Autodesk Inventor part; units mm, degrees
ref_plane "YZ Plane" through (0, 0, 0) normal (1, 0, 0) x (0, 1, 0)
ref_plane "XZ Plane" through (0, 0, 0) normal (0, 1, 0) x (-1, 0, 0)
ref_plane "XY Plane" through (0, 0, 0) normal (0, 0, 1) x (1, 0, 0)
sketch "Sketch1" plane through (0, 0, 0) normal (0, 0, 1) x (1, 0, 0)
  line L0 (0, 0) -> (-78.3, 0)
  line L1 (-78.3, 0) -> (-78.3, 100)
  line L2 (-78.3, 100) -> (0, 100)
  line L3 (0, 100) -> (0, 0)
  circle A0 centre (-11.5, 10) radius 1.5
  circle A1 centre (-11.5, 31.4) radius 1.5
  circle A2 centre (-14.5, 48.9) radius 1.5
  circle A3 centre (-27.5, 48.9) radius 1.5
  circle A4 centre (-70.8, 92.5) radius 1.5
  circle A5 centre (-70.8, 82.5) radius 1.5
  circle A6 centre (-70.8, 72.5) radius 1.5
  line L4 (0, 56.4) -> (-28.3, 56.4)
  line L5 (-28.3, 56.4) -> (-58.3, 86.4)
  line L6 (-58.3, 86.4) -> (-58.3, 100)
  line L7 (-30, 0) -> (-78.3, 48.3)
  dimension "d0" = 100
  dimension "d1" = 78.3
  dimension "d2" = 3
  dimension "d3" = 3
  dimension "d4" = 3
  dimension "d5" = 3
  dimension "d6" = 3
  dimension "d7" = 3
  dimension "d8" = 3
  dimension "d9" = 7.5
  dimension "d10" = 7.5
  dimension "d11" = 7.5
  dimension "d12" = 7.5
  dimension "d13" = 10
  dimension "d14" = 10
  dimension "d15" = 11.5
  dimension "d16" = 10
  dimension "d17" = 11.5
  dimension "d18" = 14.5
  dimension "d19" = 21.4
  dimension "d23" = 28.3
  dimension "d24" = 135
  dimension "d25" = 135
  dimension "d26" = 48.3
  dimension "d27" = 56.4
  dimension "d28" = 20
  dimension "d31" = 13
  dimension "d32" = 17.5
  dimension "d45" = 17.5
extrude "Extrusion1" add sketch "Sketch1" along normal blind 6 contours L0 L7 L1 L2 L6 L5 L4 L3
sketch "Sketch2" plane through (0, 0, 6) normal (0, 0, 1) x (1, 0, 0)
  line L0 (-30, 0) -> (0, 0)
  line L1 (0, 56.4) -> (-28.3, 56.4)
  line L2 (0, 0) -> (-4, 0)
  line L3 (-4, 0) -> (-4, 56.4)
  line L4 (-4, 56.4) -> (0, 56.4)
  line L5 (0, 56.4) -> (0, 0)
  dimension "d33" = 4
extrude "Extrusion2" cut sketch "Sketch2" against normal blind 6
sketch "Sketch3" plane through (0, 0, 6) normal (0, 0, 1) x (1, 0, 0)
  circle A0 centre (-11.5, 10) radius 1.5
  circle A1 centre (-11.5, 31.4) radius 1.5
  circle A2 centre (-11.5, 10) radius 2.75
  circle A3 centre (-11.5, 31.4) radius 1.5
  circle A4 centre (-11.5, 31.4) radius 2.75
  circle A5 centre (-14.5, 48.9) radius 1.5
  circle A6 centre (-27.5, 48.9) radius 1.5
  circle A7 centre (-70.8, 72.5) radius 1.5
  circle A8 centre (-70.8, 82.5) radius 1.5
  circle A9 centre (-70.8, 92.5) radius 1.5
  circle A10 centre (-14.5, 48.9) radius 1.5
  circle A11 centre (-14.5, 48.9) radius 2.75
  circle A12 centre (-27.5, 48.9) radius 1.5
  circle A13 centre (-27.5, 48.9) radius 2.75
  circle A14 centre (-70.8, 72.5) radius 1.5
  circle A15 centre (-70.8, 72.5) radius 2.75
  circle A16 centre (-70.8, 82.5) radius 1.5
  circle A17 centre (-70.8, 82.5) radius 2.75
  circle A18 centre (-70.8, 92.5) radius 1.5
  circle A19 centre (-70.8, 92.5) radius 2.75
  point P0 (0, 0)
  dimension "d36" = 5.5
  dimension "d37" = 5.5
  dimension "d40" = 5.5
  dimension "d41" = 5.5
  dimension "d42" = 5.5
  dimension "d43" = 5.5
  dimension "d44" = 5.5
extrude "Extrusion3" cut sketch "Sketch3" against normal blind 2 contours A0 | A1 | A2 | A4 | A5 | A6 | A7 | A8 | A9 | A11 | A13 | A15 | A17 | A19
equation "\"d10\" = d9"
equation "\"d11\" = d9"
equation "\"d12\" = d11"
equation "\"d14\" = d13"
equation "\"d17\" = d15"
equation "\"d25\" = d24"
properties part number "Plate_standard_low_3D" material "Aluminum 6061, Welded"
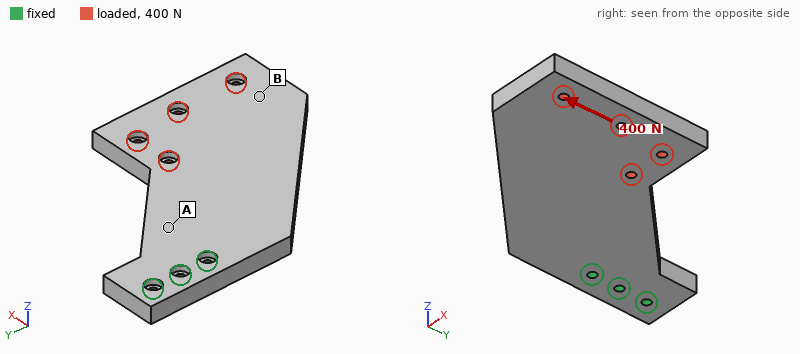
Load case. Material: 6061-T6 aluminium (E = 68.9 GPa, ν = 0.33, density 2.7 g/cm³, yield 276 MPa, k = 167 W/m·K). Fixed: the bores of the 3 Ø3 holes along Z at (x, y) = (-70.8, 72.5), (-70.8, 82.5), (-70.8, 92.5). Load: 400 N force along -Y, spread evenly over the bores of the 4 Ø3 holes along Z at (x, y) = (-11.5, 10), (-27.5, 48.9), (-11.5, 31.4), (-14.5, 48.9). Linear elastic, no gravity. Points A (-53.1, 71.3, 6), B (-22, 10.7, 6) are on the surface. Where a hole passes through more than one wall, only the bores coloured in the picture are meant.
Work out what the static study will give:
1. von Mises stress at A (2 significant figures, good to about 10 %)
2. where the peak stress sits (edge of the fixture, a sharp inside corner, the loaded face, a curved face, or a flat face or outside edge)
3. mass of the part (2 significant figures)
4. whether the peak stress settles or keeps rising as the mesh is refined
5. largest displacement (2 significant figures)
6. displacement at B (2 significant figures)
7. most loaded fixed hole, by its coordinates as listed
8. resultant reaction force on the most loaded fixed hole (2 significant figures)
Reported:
10 MPa
edge of the fixture
69 g
keeps rising
0.10 mm
0.079 mm
(-70.8, 72.5)
1.2 kN
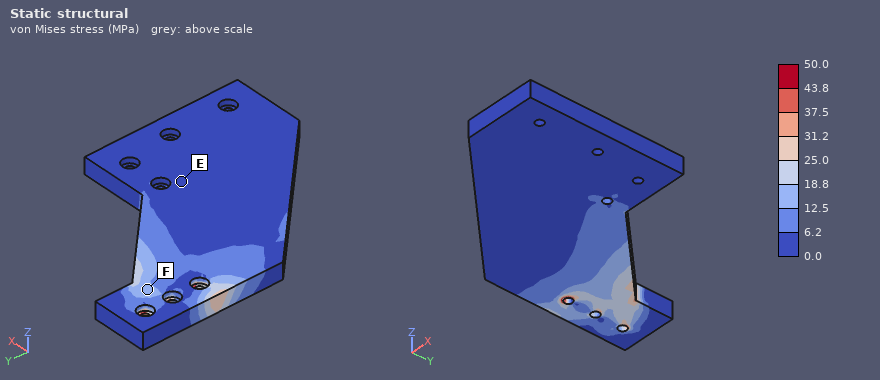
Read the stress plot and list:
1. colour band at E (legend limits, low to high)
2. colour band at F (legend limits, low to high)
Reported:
0.0 to 6.2 MPa
12.5 to 18.8 MPa
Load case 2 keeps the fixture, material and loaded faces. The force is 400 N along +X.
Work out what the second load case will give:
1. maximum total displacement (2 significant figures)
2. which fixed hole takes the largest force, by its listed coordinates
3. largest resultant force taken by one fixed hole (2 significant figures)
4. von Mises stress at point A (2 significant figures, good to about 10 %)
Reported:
68 µm
(-70.8, 72.5)
1.2 kN
7.9 MPa
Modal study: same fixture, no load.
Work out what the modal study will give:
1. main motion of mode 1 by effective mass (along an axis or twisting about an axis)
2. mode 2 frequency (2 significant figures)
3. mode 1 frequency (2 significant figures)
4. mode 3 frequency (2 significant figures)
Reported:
along Z
1800 Hz
490 Hz
1900 Hz
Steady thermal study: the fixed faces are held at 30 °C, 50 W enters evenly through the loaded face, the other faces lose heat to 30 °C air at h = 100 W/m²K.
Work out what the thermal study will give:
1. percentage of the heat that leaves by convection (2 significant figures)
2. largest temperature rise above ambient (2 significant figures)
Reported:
58 %
50 K
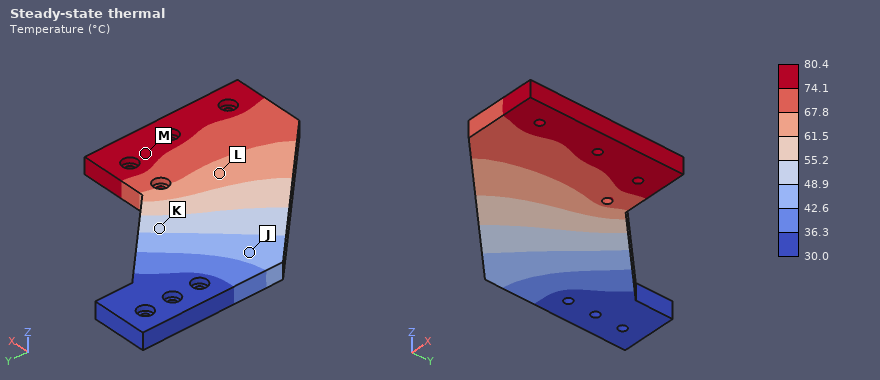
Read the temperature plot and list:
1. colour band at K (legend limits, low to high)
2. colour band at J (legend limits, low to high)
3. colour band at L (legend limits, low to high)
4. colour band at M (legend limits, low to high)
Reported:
48.9 to 55.2 °C
42.6 to 48.9 °C
61.5 to 67.8 °C
74.1 to 80.4 °C
